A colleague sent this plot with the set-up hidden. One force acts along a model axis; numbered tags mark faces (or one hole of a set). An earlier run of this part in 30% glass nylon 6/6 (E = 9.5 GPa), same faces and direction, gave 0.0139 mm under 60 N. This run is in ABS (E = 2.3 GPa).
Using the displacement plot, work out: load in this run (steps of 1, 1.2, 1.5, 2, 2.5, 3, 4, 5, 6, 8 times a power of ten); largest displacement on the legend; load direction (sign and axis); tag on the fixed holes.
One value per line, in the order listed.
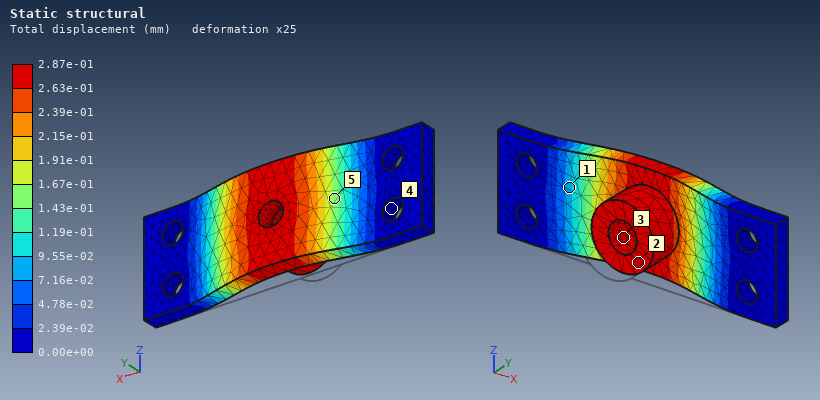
300 N
2.87e-01 mm
+Y
4
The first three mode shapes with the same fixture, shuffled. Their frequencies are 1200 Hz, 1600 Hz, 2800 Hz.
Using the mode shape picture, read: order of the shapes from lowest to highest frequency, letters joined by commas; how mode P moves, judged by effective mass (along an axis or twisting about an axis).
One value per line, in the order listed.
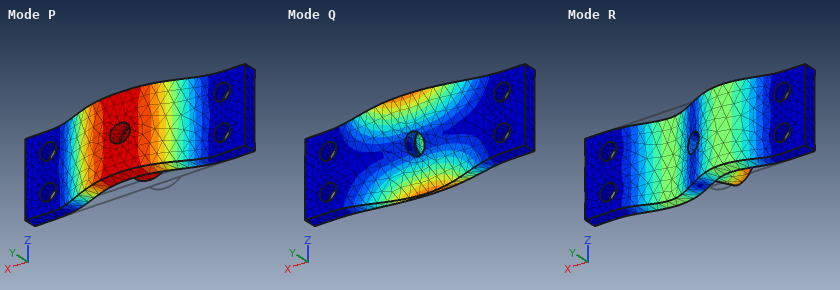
P, Q, R
along Y
